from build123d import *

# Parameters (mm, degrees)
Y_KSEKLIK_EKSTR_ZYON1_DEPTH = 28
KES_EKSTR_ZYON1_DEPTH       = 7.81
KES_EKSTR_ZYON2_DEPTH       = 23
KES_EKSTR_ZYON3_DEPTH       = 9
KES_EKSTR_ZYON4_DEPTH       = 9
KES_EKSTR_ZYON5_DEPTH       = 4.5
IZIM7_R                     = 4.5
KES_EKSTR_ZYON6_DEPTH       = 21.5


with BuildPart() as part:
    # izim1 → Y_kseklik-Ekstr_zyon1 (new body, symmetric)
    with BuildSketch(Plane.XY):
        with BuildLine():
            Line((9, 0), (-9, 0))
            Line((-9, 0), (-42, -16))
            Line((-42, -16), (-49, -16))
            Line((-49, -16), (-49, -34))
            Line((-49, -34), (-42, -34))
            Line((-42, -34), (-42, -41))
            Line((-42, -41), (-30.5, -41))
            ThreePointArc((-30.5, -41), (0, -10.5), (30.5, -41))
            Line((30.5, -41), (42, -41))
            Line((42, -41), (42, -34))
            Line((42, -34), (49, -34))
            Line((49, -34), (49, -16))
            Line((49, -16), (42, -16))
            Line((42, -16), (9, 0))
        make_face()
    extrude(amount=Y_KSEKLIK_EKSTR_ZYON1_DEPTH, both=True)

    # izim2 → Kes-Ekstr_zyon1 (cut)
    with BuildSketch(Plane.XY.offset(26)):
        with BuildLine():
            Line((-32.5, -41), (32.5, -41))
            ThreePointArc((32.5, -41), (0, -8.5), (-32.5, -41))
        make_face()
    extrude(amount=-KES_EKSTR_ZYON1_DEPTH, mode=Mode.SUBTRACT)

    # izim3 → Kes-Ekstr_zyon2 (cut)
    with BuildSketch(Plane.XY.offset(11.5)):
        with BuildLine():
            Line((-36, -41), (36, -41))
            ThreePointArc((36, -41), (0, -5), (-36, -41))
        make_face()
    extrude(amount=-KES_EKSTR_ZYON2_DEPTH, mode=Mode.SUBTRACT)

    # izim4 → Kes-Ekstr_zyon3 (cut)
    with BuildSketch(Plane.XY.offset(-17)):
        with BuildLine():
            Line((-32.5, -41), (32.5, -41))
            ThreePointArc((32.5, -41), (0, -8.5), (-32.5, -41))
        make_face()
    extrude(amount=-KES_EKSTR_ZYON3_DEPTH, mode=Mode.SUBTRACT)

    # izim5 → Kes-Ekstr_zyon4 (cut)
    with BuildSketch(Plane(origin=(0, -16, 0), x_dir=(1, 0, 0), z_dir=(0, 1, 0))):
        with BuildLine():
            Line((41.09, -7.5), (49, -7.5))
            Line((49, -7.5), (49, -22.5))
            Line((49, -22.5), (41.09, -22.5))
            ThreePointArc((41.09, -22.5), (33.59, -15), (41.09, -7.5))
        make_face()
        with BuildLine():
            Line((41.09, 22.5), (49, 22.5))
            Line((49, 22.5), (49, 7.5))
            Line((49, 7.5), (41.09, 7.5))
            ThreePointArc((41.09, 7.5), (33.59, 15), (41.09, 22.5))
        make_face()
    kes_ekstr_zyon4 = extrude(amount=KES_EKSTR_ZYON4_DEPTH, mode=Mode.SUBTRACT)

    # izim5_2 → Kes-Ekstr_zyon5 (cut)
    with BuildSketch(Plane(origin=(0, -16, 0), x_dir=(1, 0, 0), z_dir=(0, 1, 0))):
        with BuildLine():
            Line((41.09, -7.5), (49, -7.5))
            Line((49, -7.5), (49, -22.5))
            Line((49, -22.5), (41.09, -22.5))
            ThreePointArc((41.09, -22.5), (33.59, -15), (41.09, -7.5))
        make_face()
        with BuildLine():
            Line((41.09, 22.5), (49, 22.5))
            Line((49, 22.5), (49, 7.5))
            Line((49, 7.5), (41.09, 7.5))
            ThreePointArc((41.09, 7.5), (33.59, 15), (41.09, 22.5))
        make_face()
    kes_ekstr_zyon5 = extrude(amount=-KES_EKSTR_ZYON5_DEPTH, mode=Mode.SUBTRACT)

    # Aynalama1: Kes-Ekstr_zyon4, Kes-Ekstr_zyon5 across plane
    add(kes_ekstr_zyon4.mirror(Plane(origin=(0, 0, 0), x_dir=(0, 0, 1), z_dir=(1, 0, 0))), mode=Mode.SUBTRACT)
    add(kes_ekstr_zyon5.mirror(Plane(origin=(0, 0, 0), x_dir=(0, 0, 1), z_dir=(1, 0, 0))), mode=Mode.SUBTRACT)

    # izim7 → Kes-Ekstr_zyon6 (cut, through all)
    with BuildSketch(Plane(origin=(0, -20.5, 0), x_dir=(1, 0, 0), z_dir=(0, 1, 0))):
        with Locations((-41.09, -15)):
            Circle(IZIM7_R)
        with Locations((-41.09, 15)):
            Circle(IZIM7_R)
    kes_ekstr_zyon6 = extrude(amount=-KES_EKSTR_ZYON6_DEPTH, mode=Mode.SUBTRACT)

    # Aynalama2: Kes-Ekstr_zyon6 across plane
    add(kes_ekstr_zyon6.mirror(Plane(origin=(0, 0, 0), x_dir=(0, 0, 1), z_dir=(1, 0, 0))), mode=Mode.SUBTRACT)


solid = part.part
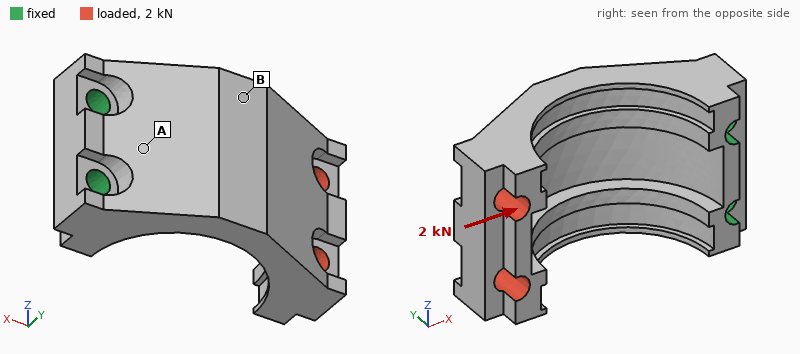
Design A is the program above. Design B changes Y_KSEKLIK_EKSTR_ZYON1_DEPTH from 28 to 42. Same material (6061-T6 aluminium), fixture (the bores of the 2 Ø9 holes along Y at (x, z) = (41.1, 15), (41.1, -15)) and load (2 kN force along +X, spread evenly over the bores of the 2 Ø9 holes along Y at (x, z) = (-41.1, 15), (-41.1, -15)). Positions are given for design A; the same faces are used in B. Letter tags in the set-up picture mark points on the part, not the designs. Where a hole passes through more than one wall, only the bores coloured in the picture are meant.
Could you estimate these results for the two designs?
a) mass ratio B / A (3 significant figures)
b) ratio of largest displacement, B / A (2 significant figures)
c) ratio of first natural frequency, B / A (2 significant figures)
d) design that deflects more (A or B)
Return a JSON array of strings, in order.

["1.68", "0.52", "1.0", "A"]
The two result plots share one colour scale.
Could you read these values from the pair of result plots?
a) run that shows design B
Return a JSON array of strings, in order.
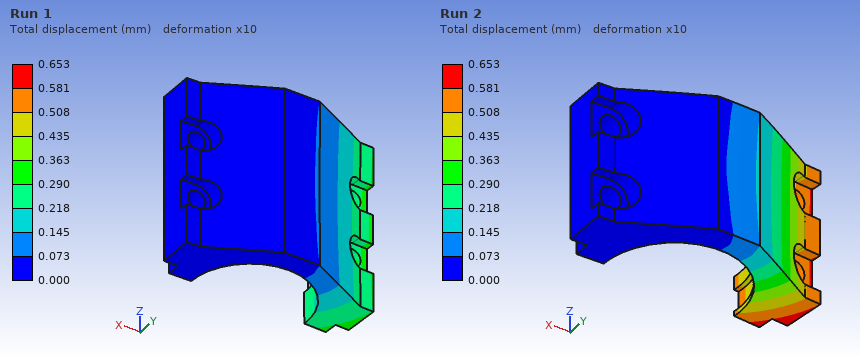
["Run 1"]
